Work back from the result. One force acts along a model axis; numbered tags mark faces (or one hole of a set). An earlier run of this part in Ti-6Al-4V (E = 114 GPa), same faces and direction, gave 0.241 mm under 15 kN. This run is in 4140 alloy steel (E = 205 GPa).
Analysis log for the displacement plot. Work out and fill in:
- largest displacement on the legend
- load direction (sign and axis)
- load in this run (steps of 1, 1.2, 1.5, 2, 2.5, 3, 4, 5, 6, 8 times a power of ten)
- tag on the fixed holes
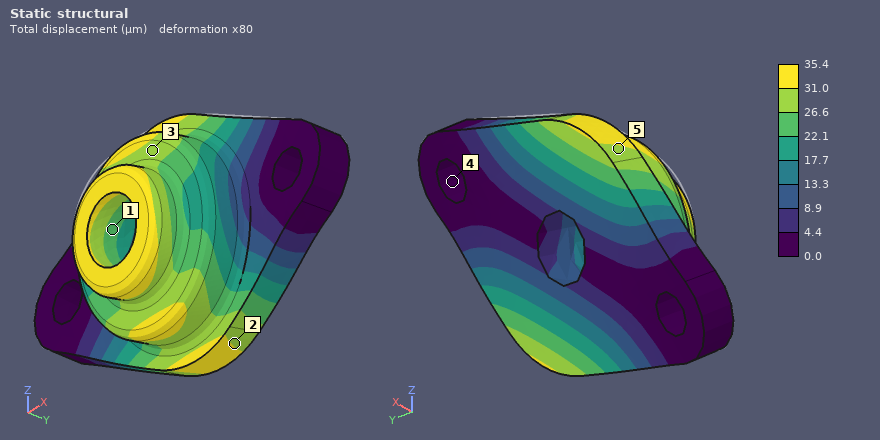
35.4 µm
-Z
4 kN
4
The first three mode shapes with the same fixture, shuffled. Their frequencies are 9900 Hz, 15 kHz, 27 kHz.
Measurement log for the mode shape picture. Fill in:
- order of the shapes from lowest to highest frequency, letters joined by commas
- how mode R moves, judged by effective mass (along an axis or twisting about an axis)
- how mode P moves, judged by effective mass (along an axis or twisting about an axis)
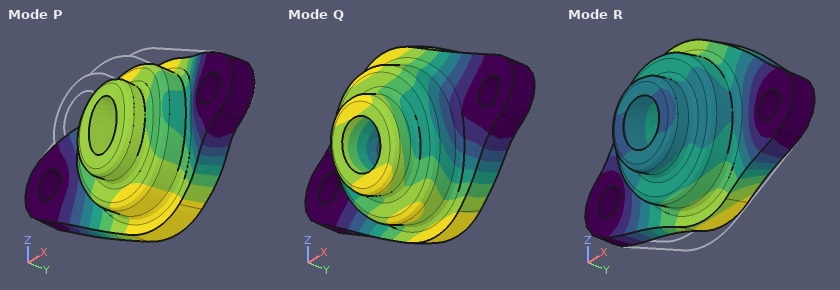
Q, P, R
along Z
along Y
